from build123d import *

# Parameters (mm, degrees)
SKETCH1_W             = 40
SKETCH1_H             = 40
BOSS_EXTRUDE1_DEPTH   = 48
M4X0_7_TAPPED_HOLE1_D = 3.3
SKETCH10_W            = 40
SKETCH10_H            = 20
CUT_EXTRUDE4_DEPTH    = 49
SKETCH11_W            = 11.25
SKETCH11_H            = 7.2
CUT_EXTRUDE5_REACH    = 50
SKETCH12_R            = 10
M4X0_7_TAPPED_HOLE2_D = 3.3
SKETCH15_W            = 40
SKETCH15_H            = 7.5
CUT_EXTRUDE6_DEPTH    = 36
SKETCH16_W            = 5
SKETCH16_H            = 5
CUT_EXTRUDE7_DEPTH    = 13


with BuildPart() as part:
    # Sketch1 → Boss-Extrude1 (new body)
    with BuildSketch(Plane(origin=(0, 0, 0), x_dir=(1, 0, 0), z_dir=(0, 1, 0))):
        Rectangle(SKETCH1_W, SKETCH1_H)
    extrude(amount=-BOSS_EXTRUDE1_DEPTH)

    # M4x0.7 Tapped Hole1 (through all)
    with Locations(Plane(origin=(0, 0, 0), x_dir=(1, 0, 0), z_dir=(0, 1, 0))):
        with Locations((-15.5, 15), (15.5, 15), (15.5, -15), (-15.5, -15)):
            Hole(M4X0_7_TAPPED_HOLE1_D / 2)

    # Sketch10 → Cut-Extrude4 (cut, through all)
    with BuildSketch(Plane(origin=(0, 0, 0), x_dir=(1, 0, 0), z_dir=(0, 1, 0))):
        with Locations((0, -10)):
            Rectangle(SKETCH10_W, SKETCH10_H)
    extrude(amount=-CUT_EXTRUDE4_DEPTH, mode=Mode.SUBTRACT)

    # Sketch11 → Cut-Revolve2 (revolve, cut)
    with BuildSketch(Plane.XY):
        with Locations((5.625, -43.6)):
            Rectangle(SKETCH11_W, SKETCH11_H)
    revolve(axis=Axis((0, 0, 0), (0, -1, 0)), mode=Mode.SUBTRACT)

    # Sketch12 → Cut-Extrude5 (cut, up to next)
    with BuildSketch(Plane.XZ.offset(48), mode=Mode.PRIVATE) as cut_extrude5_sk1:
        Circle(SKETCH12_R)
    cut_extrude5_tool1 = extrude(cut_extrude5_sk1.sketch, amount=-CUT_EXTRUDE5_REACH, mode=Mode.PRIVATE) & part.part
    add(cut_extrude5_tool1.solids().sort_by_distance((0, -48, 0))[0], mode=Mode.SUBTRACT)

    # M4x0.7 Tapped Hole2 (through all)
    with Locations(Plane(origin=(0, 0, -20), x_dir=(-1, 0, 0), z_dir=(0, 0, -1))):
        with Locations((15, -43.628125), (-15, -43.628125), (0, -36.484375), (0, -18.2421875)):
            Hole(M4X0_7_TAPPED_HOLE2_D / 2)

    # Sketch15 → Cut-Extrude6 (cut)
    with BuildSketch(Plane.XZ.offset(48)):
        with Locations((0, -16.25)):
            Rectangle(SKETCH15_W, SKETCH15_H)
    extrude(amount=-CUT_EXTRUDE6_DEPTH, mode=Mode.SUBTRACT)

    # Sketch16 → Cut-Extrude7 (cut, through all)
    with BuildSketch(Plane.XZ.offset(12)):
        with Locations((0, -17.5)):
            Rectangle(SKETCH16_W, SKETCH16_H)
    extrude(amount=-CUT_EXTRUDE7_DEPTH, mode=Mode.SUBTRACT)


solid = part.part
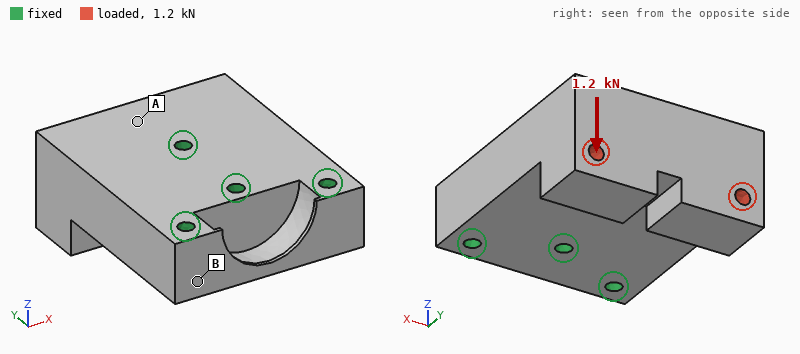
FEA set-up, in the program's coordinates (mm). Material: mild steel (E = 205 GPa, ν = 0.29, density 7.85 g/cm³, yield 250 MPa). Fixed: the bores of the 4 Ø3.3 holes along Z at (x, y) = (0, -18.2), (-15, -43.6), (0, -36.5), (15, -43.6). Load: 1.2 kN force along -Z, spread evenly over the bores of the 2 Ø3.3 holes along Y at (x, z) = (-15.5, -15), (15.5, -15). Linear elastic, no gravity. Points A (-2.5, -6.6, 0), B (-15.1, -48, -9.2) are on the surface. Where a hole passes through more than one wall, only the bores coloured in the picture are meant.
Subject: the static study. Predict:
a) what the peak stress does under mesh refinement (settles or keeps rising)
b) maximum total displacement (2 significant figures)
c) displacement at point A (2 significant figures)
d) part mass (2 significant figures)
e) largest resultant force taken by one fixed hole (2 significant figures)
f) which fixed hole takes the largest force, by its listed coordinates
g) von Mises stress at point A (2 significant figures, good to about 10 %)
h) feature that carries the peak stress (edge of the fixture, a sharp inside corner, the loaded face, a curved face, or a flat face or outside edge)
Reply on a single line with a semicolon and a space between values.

keeps rising; 4.1 µm; 1.9 µm; 200 g; 1.4 kN; (0, -18.2); 7.1 MPa; edge of the fixture
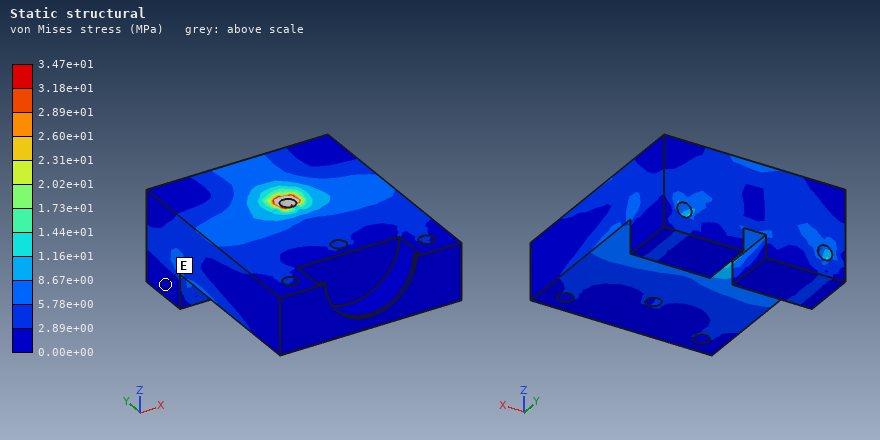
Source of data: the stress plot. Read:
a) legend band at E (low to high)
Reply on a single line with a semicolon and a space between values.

0.00e+00 to 2.89e+00 MPa
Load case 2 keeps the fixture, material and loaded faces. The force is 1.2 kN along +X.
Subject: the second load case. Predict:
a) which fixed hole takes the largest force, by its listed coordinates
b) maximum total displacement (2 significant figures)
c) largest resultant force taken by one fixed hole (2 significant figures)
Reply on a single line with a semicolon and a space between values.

(0, -18.2); 3.3 µm; 1.4 kN
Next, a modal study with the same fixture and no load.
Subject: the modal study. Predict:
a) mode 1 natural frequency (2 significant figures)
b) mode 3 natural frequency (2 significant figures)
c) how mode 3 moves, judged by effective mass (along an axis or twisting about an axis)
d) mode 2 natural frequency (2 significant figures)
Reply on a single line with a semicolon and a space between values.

12 kHz; 19 kHz; along X; 13 kHz
